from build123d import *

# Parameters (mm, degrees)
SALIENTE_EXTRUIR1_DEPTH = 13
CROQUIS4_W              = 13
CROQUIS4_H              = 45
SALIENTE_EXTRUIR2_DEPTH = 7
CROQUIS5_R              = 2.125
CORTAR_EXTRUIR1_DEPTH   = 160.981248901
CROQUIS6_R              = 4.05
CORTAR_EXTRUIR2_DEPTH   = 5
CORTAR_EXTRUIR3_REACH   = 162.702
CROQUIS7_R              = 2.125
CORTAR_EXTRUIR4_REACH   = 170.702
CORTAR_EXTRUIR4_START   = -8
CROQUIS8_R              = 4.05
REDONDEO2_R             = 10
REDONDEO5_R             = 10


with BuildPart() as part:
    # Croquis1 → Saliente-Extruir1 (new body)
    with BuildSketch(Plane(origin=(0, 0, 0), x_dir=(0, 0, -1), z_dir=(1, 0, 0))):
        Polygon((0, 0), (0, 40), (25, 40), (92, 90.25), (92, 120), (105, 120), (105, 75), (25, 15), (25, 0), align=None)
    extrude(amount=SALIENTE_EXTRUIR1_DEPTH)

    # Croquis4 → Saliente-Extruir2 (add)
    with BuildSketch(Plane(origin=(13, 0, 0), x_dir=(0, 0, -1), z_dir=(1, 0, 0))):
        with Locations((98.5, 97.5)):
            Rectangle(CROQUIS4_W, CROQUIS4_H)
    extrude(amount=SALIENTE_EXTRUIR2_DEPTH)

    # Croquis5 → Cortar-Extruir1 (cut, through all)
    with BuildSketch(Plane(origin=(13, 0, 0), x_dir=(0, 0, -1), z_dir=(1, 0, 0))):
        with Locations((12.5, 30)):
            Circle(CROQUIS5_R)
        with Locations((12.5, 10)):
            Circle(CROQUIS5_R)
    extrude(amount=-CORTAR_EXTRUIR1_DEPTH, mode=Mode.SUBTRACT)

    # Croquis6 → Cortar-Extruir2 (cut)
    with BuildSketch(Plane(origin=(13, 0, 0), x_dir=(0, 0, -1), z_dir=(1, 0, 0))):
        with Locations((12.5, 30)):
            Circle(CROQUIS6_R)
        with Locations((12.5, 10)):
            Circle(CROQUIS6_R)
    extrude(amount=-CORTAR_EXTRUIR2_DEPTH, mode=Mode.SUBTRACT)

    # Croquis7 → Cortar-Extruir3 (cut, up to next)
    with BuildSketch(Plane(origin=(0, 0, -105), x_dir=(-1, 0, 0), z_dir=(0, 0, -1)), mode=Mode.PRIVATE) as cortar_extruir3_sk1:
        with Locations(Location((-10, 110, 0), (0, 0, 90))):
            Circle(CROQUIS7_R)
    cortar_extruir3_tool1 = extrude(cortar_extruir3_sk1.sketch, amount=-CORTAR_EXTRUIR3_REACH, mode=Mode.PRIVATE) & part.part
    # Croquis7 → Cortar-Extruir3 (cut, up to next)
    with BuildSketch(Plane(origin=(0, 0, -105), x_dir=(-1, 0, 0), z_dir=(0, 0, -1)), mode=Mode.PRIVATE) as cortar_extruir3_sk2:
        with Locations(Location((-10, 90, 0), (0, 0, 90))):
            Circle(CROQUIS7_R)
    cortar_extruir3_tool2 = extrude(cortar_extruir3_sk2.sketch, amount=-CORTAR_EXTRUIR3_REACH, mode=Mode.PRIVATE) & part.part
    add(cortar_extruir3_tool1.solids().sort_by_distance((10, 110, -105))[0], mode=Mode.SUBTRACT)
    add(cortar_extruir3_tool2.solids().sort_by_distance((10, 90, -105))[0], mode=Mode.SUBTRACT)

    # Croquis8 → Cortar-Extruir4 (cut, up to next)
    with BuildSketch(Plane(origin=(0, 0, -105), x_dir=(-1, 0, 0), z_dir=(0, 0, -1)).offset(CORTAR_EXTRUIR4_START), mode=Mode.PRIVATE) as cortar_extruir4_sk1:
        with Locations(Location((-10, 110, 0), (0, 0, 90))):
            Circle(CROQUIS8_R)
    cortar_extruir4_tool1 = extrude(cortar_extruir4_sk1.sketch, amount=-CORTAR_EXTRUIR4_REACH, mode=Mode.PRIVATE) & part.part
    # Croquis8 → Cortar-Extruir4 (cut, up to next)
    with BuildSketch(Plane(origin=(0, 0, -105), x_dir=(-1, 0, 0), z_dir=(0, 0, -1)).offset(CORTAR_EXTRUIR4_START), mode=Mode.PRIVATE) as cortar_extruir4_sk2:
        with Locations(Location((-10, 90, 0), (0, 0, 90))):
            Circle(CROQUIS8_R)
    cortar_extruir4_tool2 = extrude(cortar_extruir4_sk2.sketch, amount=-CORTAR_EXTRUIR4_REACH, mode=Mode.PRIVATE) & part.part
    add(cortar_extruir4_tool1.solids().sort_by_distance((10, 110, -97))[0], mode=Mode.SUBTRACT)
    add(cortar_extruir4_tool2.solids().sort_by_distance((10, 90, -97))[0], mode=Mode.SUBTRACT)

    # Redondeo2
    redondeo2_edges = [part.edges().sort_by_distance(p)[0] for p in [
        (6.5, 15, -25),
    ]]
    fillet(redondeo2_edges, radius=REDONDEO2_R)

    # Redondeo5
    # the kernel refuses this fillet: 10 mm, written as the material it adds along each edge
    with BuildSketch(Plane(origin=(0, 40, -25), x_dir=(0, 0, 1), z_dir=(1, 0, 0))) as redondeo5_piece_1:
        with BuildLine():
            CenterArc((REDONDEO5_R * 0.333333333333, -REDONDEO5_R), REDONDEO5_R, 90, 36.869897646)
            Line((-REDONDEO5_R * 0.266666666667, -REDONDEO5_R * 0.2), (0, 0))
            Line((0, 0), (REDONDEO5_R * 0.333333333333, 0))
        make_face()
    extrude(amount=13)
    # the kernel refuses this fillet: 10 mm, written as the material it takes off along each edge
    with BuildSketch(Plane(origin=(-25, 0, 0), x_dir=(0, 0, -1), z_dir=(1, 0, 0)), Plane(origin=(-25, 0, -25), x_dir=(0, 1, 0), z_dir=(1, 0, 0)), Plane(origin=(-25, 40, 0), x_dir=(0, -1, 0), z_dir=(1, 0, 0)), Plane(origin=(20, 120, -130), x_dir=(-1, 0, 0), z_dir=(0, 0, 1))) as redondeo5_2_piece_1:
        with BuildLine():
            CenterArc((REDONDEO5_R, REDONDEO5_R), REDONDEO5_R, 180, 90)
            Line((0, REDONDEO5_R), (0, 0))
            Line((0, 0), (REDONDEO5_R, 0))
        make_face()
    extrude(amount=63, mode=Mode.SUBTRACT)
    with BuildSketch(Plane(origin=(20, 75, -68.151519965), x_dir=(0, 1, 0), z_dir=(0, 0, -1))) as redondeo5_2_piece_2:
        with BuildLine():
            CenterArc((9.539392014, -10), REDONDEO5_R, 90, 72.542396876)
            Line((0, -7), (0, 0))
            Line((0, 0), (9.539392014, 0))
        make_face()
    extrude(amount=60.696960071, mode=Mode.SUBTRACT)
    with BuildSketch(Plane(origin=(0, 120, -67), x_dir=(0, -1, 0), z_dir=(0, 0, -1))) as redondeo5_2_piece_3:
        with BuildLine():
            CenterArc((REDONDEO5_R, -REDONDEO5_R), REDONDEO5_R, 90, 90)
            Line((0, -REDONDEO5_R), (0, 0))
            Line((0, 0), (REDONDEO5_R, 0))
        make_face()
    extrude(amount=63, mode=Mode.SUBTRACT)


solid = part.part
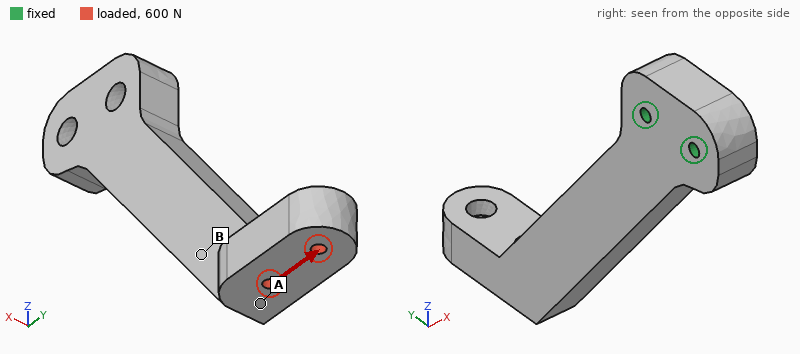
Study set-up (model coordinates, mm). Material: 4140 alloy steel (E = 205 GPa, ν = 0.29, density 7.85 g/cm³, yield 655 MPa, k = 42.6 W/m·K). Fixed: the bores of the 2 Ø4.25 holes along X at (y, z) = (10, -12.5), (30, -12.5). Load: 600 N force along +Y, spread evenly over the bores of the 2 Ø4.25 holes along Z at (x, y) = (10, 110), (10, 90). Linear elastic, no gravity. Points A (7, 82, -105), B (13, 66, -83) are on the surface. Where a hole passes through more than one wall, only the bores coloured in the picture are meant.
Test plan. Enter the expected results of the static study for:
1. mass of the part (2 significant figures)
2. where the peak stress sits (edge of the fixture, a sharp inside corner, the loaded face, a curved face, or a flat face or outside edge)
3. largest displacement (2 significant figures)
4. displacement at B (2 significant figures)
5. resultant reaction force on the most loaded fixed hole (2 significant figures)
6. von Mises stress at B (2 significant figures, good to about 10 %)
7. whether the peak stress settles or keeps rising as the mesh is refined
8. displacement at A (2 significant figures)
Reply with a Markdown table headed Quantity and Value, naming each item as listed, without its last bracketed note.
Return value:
| Quantity | Value |
|---|---|
| mass of the part | 350 g |
| where the peak stress sits | edge of the fixture |
| largest displacement | 0.14 mm |
| displacement at B | 0.063 mm |
| resultant reaction force on the most loaded fixed hole | 2.6 kN |
| von Mises stress at B | 12 MPa |
| whether the peak stress settles or keeps rising as the mesh is refined | keeps rising |
| displacement at A | 0.099 mm |
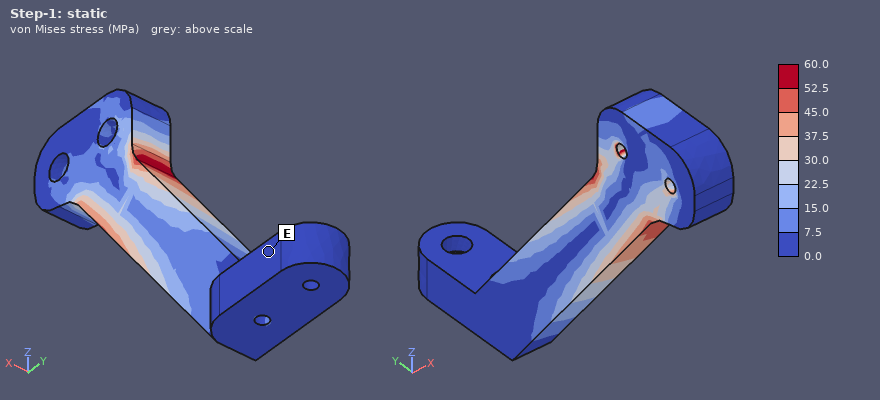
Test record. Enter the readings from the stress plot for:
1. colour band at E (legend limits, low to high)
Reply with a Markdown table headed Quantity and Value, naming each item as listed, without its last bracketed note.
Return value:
| Quantity | Value |
|---|---|
| colour band at E | 0.0 to 7.5 MPa |
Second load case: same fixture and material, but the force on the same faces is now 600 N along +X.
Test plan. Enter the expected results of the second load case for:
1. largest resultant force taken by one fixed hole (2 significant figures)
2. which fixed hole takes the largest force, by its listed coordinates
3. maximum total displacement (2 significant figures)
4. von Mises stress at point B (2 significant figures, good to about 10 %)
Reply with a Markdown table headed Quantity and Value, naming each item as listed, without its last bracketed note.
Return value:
| Quantity | Value |
|---|---|
| largest resultant force taken by one fixed hole | 2.2 kN |
| which fixed hole takes the largest force, by its listed coordinates | (30, -12.5) |
| maximum total displacement | 0.54 mm |
| von Mises stress at point B | 40 MPa |
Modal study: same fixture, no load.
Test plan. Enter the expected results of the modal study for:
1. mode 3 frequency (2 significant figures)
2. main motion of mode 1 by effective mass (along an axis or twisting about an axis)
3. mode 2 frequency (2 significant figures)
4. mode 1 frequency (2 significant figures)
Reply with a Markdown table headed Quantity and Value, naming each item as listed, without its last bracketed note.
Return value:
| Quantity | Value |
|---|---|
| mode 3 frequency | 2700 Hz |
| main motion of mode 1 by effective mass | along X |
| mode 2 frequency | 970 Hz |
| mode 1 frequency | 580 Hz |
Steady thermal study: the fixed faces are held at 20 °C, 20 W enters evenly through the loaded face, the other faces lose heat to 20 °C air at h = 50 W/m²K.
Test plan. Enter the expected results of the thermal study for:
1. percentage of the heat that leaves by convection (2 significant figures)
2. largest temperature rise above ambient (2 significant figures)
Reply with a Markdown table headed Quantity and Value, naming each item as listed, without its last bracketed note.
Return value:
| Quantity | Value |
|---|---|
| percentage of the heat that leaves by convection | 82 % |
| largest temperature rise above ambient | 76 K |
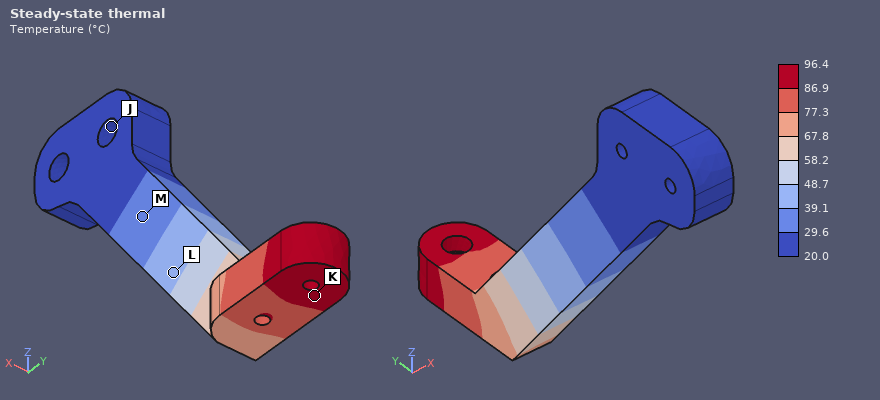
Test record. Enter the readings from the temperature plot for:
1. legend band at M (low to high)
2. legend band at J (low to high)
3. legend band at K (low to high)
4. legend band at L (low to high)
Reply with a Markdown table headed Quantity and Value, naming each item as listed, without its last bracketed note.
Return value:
| Quantity | Value |
|---|---|
| legend band at M | 29.6 to 39.1 °C |
| legend band at J | 20.0 to 29.6 °C |
| legend band at K | 86.9 to 96.4 °C |
| legend band at L | 39.1 to 48.7 °C |
